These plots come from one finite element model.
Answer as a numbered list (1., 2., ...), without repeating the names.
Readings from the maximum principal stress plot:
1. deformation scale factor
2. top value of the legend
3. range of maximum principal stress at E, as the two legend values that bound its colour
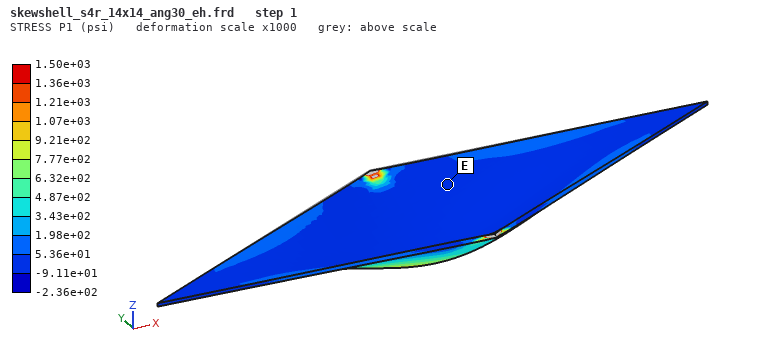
1. 1000
2. 1.50e+03 psi
3. -9.11e+01 to 5.36e+01 psi
